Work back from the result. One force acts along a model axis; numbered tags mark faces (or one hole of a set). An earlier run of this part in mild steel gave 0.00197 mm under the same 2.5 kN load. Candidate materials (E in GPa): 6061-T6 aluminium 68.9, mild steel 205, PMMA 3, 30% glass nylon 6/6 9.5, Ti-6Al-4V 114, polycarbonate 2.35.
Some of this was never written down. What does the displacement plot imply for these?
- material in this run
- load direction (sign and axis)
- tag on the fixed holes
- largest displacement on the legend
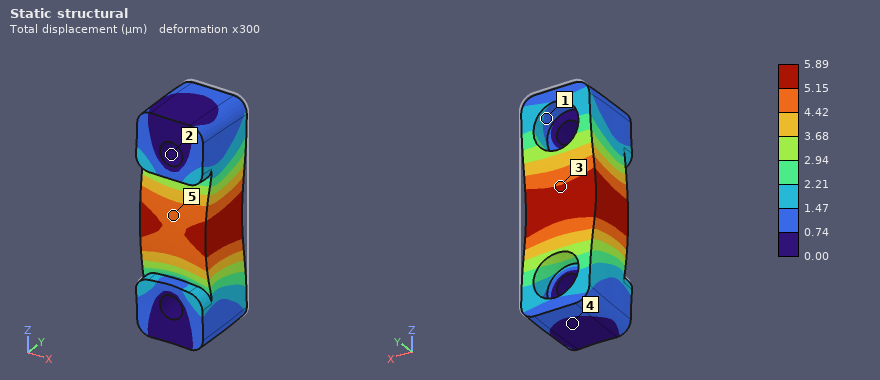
6061-T6 aluminium
-Y
2
5.89 µm
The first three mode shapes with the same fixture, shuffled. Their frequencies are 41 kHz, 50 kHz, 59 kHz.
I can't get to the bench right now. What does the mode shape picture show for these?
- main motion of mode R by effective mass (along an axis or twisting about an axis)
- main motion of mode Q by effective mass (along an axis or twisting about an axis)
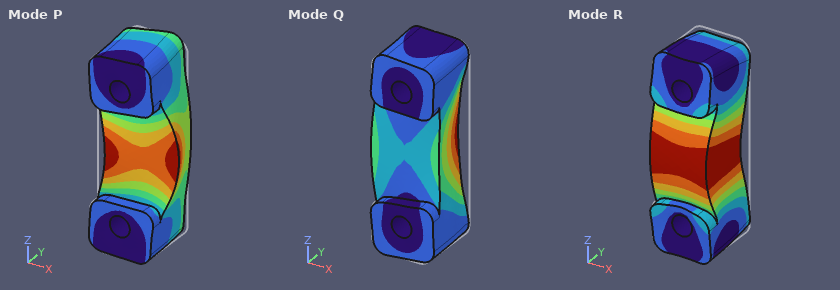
along Y
along X
